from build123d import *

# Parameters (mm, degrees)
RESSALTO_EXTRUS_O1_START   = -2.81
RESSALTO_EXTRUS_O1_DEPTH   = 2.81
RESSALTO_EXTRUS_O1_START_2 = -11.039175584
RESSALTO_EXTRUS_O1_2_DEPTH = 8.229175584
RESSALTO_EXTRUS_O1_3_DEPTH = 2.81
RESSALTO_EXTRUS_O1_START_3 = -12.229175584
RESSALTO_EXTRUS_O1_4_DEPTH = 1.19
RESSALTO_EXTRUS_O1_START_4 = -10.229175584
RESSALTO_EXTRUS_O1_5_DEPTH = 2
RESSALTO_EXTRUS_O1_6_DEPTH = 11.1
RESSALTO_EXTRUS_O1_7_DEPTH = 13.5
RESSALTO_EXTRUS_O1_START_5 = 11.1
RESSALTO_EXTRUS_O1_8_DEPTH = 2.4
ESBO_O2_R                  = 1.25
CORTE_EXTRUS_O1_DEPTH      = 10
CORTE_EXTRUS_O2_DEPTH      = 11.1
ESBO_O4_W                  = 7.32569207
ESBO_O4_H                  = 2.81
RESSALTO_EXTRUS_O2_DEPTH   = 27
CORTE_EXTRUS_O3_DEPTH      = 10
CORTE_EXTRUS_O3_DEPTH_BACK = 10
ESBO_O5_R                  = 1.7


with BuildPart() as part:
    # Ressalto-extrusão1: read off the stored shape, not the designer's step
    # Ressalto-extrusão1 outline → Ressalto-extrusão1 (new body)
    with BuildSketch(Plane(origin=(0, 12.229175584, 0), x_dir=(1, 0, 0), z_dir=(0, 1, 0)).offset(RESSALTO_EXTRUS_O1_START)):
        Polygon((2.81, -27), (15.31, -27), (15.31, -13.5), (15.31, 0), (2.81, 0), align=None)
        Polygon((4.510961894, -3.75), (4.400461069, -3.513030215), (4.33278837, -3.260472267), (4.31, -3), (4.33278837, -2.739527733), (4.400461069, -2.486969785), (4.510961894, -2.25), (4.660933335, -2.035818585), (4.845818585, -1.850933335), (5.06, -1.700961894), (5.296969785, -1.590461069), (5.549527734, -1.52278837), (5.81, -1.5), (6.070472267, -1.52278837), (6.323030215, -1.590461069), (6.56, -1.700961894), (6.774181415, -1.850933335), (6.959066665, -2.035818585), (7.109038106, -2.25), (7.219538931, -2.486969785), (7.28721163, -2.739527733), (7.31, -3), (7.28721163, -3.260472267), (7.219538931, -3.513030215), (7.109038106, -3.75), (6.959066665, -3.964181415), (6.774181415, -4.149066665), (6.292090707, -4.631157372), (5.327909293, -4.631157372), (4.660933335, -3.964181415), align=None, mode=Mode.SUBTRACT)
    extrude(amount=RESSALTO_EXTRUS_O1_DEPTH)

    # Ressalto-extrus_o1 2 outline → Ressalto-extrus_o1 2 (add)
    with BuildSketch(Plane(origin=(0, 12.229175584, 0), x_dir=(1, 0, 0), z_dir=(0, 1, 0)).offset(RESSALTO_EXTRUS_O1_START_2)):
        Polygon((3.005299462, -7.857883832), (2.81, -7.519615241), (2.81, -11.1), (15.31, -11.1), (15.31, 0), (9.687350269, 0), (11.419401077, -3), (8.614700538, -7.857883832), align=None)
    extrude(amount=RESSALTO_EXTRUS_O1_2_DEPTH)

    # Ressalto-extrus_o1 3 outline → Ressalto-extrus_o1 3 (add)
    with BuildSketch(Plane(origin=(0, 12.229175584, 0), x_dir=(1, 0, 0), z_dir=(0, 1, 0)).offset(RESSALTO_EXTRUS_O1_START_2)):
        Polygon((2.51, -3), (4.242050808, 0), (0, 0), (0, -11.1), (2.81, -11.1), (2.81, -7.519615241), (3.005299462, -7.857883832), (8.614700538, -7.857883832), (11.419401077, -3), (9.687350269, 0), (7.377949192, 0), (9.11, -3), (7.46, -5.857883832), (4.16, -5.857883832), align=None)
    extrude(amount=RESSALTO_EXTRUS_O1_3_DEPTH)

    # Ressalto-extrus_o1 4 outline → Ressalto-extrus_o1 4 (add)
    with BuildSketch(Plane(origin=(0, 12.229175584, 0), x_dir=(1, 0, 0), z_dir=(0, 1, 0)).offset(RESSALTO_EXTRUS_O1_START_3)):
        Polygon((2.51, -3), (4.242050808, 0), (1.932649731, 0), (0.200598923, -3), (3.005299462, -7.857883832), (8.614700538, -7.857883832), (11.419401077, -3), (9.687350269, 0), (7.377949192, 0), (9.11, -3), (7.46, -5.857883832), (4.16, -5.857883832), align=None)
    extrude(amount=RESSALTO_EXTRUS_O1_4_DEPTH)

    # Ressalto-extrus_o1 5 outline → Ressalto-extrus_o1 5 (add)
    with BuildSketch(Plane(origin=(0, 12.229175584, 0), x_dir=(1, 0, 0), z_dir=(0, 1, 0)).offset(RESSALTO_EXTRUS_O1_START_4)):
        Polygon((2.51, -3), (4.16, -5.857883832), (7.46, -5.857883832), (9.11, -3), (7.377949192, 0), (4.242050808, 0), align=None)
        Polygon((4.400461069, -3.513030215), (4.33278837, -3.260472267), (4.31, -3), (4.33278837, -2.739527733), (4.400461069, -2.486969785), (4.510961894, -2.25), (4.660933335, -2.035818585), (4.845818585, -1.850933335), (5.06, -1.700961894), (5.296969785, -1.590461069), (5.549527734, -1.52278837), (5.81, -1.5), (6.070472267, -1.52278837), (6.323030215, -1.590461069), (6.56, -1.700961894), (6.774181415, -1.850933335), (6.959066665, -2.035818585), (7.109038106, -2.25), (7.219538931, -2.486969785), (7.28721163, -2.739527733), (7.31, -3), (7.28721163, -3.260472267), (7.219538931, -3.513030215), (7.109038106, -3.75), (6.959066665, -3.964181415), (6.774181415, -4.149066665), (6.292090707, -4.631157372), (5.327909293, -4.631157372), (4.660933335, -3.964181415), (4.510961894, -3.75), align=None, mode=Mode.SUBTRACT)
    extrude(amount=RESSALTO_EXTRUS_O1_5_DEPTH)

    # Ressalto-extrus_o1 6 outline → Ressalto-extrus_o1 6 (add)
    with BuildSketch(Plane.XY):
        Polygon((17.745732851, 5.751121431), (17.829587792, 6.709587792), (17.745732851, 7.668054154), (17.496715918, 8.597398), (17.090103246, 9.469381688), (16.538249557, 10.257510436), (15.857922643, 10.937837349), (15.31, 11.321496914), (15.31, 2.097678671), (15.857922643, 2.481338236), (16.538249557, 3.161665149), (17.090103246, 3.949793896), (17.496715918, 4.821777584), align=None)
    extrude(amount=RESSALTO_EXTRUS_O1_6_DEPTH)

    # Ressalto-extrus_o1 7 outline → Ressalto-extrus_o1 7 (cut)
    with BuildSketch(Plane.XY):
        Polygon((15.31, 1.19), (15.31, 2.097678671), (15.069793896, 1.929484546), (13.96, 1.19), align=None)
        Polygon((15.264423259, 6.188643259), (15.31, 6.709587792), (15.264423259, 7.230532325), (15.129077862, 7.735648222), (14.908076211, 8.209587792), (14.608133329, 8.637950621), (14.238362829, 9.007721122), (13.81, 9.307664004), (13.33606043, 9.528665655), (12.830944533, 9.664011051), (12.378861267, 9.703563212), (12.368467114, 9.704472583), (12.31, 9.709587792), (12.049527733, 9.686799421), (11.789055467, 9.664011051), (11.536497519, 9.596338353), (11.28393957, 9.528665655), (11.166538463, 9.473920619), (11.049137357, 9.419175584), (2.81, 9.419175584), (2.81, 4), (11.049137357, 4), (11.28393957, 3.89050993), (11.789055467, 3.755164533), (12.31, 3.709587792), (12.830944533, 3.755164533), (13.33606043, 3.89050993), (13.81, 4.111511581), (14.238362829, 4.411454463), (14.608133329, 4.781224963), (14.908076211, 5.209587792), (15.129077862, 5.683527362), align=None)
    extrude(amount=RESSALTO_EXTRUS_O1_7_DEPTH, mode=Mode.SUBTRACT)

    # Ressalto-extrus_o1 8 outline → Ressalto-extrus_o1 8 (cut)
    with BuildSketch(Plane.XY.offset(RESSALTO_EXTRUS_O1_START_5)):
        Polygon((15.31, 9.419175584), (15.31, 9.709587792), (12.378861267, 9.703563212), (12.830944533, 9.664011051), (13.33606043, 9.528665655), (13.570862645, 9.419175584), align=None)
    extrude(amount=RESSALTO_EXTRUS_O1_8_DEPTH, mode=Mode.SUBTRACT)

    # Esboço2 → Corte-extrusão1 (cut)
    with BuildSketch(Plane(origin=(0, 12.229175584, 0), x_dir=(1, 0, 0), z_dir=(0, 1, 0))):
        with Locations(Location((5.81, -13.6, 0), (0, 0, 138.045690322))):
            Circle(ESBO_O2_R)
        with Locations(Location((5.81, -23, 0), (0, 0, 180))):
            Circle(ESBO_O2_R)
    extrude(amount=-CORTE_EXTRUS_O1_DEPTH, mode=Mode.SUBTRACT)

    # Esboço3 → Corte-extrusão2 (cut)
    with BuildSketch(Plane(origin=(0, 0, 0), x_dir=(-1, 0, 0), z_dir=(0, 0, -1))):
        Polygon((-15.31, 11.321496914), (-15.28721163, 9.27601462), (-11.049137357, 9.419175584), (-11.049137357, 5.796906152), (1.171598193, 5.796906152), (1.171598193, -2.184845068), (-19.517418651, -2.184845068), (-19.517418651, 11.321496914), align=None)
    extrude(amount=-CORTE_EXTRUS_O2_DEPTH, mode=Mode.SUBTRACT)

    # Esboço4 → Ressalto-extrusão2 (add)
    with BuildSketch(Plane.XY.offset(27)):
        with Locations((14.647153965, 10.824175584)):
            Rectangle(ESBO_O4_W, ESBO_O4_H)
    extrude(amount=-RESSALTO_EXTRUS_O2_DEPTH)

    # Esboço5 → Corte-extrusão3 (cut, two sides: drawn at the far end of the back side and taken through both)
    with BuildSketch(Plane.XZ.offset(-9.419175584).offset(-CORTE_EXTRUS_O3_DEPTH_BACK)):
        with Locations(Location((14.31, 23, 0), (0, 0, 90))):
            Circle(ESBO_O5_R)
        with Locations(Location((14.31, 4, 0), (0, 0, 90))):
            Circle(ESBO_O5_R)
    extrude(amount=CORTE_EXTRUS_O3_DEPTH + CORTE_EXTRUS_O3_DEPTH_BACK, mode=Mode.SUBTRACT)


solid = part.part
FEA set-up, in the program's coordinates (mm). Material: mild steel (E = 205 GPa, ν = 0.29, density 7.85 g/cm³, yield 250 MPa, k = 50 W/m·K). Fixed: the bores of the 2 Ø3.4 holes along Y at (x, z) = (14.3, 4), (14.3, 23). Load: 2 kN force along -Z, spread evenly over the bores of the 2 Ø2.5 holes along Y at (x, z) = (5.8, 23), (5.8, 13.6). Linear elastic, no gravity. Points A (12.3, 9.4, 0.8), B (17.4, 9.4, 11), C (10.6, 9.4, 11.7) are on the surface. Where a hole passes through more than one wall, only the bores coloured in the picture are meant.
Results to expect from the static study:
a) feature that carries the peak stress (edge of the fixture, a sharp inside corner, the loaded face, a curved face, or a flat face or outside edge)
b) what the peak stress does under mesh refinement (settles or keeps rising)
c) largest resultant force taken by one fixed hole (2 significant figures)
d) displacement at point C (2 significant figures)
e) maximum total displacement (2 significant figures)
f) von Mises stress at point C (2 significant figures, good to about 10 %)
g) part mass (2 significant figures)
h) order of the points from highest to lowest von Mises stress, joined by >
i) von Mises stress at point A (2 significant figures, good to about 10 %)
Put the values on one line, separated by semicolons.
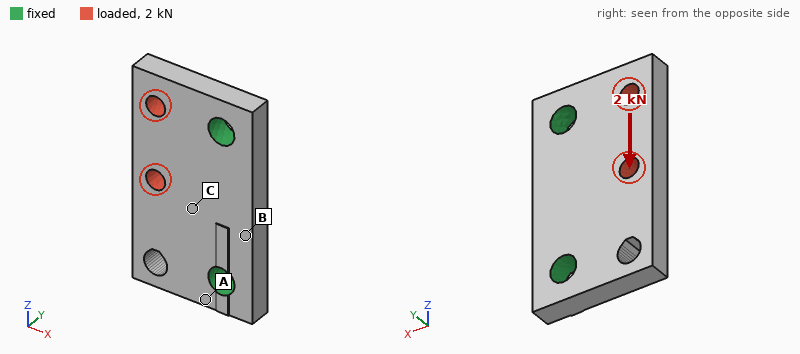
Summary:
edge of the fixture; keeps rising; 1.3 kN; 1.7 µm; 6.8 µm; 55 MPa; 8.5 g; C > A > B; 29 MPa
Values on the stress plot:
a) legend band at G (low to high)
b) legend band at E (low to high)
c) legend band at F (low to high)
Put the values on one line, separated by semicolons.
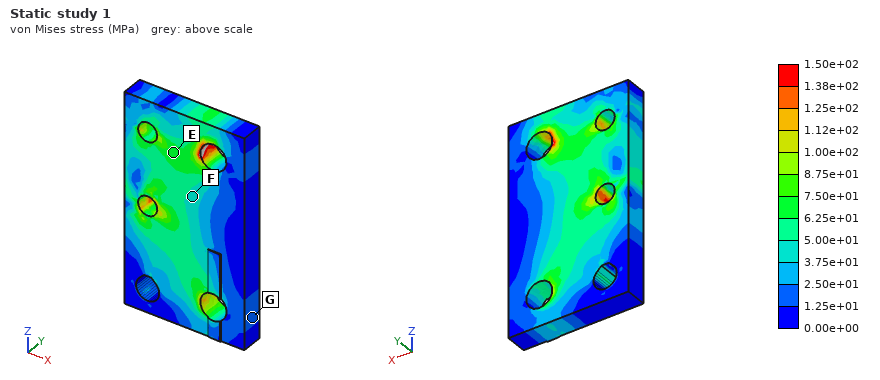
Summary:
1.25e+01 to 2.50e+01 MPa; 6.25e+01 to 7.50e+01 MPa; 3.75e+01 to 5.00e+01 MPa
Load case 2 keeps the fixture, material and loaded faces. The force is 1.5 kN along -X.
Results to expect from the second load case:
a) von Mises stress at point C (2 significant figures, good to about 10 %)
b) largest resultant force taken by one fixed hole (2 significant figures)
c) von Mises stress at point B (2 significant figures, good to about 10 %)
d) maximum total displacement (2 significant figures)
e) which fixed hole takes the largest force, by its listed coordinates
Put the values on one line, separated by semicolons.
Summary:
20 MPa; 1.1 kN; 12 MPa; 2.6 µm; (14.3, 23)
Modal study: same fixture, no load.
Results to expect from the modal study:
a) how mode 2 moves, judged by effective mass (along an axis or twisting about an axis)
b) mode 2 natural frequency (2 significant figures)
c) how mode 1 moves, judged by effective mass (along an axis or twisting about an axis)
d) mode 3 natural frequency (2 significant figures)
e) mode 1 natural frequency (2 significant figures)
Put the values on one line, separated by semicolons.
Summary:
twisting about X; 26 kHz; along Y; 36 kHz; 17 kHz
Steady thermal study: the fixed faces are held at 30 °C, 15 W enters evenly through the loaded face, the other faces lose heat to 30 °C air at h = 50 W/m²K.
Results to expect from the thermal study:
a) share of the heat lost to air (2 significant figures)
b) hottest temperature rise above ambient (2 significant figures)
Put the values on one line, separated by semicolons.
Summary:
6.6 %; 58 K
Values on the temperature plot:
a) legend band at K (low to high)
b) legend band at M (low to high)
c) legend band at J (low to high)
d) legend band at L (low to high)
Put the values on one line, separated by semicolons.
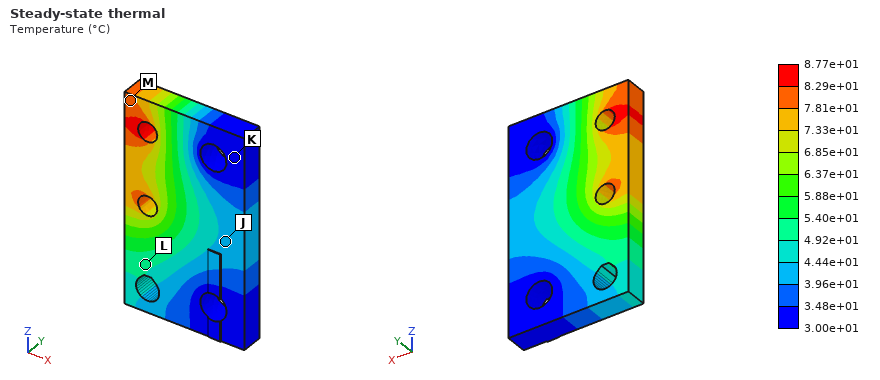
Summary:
3.00e+01 to 3.48e+01 °C; 7.81e+01 to 8.29e+01 °C; 3.96e+01 to 4.44e+01 °C; 4.92e+01 to 5.40e+01 °C
